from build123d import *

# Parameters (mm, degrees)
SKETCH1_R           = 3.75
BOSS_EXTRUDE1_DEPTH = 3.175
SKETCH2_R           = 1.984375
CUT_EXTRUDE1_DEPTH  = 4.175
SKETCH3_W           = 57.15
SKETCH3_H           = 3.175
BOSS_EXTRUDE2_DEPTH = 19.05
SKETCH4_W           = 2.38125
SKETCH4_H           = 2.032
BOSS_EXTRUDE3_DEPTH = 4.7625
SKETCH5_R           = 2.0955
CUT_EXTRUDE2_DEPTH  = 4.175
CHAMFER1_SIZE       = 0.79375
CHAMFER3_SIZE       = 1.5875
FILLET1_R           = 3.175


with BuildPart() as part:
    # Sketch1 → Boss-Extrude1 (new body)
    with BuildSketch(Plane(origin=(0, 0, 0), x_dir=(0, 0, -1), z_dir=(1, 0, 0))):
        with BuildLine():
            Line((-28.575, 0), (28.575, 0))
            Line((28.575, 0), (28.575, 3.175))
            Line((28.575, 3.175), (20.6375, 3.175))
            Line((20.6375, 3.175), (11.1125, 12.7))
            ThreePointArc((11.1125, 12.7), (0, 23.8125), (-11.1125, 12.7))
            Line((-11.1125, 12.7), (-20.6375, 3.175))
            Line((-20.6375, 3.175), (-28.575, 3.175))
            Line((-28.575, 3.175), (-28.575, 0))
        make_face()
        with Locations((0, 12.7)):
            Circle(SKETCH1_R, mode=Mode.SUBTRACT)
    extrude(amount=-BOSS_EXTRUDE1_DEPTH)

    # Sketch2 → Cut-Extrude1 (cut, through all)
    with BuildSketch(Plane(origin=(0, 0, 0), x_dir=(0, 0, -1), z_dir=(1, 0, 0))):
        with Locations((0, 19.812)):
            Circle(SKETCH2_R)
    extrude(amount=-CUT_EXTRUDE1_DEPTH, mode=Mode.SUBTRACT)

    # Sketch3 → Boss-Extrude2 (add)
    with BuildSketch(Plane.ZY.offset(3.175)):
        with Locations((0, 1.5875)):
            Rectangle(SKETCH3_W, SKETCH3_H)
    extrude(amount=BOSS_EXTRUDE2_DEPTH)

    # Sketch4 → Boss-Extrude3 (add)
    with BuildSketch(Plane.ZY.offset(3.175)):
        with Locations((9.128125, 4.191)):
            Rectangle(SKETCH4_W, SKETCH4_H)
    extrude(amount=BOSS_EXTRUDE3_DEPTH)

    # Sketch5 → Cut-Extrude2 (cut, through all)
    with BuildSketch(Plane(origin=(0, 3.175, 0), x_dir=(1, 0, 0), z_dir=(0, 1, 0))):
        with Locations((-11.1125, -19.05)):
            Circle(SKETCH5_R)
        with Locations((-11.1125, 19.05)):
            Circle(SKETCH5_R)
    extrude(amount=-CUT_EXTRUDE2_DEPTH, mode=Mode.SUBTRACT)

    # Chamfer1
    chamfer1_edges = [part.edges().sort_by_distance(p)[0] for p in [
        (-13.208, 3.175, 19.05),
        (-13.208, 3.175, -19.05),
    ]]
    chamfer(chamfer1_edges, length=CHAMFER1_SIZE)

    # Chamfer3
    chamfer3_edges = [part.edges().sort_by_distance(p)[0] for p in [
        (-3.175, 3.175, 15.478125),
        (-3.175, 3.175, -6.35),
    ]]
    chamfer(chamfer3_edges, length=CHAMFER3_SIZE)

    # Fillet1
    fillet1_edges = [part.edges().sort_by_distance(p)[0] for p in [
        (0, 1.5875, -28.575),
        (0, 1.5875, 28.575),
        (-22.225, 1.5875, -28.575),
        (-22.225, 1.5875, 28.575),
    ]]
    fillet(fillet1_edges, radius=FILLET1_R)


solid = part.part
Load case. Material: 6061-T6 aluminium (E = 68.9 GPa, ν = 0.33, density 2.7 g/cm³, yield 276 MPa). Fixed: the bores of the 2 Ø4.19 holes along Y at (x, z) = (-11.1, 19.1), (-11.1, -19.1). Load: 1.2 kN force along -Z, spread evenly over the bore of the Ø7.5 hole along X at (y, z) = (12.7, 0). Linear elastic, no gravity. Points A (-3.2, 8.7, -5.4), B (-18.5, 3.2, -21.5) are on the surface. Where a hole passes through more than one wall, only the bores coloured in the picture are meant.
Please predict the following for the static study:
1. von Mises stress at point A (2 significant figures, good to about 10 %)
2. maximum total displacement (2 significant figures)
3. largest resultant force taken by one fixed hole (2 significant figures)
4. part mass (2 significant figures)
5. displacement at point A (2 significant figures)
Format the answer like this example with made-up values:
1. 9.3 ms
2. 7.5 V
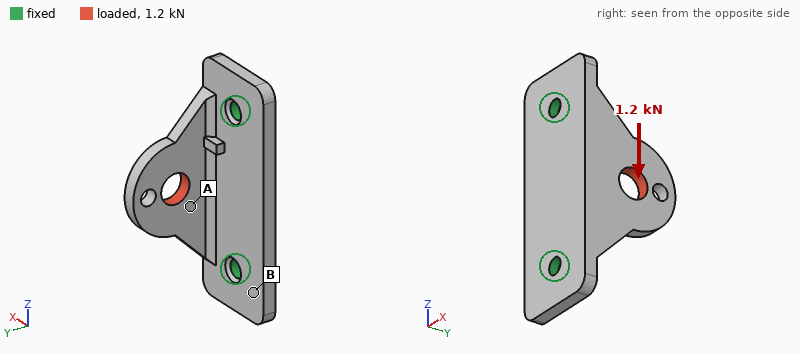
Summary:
1. 29 MPa
2. 44 µm
3. 750 N
4. 15 g
5. 18 µm
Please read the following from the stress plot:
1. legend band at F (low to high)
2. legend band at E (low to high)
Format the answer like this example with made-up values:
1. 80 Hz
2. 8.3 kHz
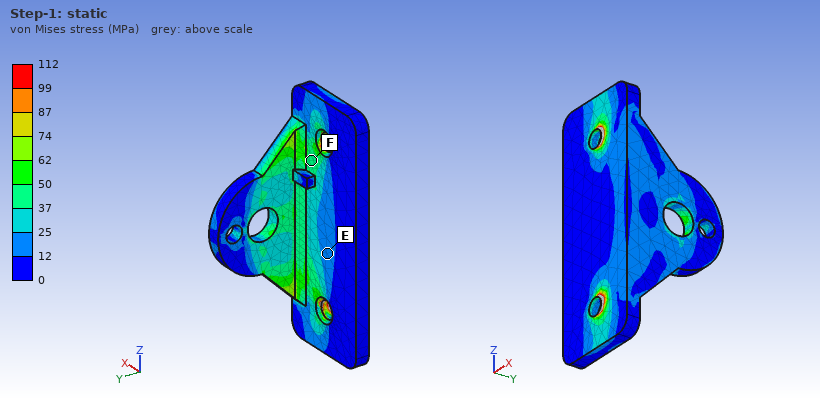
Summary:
1. 37 to 50 MPa
2. 12 to 25 MPa
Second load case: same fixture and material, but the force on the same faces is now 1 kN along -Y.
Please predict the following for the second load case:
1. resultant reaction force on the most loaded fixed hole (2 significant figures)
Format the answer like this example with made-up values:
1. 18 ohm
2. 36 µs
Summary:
1. 570 N
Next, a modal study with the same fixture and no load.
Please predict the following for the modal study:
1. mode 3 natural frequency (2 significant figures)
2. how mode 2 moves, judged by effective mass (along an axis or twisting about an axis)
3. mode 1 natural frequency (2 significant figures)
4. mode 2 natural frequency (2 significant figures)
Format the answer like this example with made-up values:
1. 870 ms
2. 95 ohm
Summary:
1. 12 kHz
2. along Y
3. 4900 Hz
4. 11 kHz
